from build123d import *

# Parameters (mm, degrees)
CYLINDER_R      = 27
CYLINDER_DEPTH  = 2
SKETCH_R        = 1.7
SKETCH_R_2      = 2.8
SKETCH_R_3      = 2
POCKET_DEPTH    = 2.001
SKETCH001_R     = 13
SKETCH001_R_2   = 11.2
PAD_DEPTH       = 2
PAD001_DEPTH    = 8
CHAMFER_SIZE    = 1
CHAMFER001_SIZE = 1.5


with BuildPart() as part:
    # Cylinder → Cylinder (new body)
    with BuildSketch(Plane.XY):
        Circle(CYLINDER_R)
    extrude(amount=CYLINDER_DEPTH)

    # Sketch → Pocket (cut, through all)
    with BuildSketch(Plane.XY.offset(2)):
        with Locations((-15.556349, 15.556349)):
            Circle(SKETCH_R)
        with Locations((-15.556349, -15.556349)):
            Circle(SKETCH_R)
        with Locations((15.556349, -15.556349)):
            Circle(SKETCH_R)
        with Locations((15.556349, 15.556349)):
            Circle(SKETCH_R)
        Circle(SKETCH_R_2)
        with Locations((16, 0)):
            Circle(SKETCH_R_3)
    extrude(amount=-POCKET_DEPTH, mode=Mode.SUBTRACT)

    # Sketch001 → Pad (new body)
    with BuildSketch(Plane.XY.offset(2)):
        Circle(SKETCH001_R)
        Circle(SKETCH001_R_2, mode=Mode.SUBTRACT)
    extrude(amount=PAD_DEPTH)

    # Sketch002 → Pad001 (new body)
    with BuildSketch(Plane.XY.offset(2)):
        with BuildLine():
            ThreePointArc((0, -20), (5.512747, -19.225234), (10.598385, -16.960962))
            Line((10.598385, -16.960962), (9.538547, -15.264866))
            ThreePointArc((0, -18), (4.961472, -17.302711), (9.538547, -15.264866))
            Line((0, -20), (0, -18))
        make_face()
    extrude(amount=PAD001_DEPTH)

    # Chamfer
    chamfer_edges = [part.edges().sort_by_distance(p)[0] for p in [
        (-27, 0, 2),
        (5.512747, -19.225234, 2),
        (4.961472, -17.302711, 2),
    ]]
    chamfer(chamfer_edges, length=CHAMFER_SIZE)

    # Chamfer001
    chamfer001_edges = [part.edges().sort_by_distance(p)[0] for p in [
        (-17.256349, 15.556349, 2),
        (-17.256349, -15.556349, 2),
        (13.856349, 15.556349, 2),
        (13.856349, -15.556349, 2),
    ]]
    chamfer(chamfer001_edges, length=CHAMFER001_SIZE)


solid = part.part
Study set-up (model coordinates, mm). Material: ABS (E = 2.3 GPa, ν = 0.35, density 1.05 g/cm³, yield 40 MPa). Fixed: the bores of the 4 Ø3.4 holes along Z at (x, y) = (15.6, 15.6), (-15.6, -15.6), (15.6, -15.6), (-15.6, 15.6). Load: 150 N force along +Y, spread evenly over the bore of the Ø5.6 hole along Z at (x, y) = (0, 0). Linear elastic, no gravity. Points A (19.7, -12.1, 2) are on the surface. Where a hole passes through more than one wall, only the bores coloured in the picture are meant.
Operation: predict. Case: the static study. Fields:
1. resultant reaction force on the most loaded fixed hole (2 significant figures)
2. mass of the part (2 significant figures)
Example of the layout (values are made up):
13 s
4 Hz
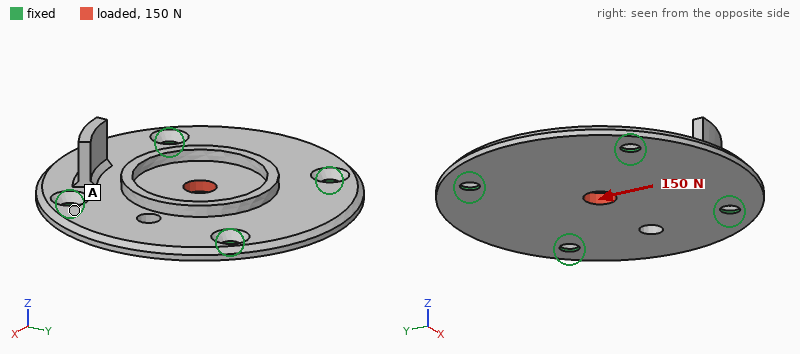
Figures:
39 N
5.0 g
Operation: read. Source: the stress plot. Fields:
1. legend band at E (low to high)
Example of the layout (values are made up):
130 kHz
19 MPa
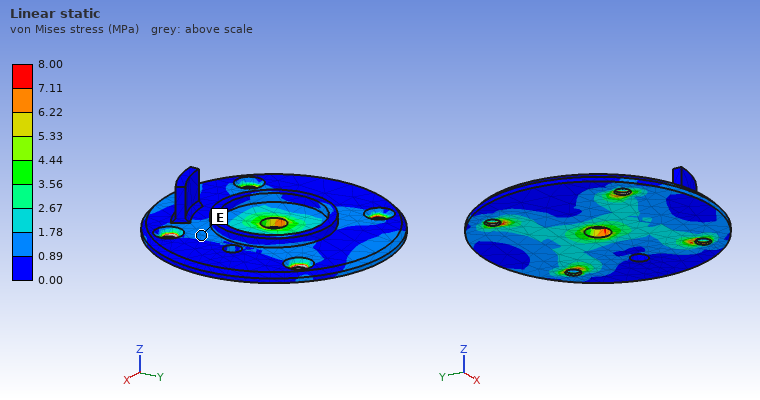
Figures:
0.89 to 1.78 MPa
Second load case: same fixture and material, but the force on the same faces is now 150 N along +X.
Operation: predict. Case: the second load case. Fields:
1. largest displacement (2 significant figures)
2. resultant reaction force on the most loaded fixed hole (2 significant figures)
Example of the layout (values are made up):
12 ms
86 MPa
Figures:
28 µm
39 N
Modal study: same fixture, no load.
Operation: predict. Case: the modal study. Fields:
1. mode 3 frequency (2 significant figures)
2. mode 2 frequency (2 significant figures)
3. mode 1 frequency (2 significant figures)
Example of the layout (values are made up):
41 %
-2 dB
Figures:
2200 Hz
2200 Hz
2000 Hz
